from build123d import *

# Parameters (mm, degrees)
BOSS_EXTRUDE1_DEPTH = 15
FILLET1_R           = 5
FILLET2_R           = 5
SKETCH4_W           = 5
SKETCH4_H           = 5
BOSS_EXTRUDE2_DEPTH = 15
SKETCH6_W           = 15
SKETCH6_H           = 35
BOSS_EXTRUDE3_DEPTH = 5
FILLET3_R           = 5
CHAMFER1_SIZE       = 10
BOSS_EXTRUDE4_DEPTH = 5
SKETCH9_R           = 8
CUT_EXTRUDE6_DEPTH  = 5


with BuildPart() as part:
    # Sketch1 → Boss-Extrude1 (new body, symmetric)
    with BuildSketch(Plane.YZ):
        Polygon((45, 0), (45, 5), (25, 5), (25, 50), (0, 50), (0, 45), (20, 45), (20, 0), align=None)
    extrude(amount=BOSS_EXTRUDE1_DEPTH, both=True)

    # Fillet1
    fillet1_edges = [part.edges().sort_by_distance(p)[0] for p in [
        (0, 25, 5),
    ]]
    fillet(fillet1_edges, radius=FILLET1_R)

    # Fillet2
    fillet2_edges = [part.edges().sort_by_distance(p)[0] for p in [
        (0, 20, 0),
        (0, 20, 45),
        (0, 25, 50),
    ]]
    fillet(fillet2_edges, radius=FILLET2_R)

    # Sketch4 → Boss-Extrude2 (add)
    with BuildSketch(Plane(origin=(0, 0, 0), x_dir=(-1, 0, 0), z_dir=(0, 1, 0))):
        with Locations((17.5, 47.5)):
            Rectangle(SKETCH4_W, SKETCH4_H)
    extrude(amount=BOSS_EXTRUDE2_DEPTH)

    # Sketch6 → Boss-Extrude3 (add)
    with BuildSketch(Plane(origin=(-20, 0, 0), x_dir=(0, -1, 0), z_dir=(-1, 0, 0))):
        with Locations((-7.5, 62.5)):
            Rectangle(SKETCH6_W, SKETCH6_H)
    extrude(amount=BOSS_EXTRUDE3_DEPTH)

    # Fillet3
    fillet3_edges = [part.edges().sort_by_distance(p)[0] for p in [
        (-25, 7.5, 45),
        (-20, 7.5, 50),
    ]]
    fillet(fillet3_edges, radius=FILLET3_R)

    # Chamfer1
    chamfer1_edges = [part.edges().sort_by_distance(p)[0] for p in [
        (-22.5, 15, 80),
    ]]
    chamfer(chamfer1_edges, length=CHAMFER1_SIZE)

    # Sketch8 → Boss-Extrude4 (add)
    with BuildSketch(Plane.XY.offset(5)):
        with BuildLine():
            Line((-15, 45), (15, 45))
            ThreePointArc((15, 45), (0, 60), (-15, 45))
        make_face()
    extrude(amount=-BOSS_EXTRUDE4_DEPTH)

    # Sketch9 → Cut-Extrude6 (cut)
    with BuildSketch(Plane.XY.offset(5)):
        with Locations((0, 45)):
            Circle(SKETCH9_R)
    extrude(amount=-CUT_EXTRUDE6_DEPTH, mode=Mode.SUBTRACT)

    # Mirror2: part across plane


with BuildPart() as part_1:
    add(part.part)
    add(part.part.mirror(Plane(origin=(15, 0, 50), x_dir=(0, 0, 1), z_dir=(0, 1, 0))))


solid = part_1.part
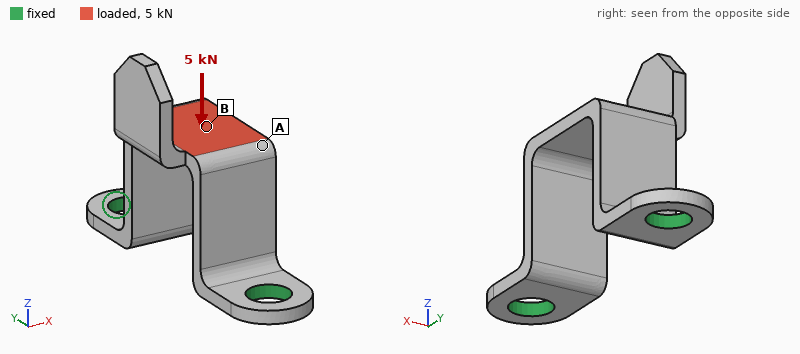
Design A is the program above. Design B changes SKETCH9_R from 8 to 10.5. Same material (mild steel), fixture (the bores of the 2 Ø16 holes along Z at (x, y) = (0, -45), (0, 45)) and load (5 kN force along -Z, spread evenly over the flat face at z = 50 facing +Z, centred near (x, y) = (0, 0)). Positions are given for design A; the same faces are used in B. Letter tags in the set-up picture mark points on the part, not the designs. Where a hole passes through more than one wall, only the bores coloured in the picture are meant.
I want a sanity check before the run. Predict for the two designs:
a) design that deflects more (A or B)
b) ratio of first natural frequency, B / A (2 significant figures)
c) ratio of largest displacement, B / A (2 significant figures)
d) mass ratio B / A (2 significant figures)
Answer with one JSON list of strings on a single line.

["A", "1.2", "0.87", "0.96"]
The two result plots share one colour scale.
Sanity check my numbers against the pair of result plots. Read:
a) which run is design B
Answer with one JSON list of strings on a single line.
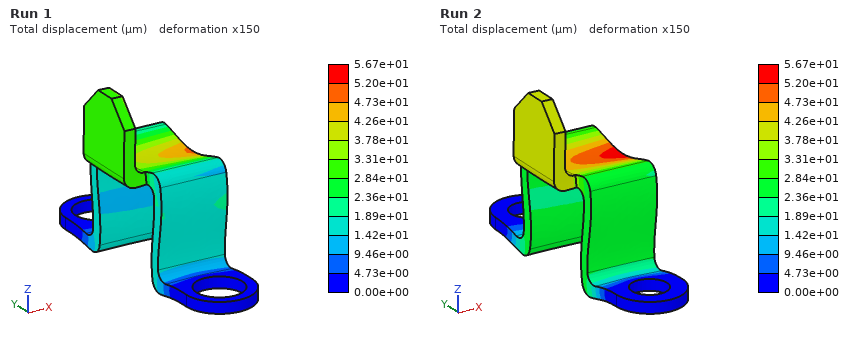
["Run 1"]
